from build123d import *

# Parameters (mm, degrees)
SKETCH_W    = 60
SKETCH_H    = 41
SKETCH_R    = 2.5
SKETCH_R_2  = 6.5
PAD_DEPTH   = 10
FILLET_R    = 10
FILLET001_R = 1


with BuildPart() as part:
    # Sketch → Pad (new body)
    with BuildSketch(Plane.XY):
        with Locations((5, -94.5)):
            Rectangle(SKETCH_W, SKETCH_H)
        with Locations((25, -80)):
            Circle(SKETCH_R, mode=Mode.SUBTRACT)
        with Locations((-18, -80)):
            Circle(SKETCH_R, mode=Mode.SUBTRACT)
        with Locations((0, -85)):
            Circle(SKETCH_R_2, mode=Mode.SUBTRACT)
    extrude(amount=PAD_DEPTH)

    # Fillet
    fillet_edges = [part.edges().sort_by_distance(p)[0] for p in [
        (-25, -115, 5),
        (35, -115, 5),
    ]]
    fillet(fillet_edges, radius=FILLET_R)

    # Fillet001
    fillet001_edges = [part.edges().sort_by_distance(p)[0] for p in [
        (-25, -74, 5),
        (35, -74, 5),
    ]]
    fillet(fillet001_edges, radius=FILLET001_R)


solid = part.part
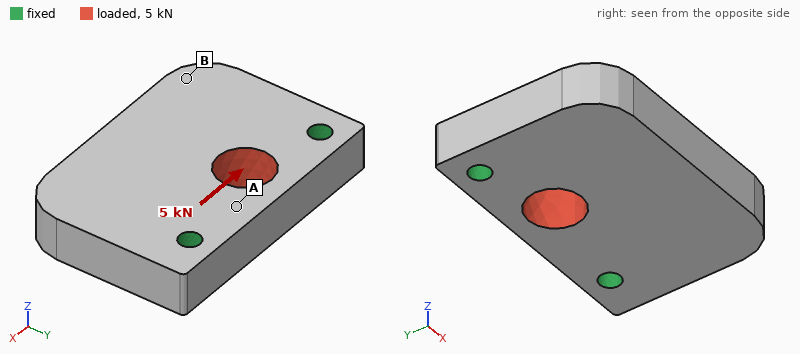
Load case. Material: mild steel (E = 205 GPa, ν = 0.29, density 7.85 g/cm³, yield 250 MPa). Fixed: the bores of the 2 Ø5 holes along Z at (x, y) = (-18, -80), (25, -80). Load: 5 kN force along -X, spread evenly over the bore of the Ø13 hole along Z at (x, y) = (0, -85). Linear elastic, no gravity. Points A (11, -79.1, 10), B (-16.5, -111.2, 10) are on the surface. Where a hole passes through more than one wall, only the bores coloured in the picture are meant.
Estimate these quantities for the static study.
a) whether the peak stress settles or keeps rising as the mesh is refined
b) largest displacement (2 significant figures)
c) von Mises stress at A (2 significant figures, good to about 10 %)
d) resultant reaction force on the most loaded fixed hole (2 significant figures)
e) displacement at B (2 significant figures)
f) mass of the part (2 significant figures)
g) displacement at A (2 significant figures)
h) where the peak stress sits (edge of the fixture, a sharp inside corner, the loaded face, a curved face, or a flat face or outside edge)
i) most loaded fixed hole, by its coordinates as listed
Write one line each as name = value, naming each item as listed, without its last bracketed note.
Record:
whether the peak stress settles or keeps rising as the mesh is refined = keeps rising
largest displacement = 2.1 µm
von Mises stress at A = 12 MPa
resultant reaction force on the most loaded fixed hole = 2.7 kN
displacement at B = 1.6 µm
mass of the part = 180 g
displacement at A = 0.88 µm
where the peak stress sits = edge of the fixture
most loaded fixed hole, by its coordinates as listed = (-18, -80)
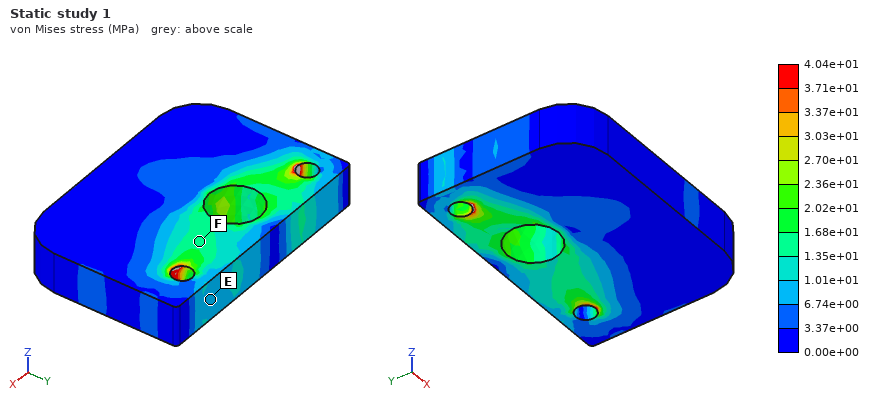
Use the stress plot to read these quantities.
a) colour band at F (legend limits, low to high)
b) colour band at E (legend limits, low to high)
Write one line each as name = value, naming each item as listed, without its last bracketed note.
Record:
colour band at F = 1.35e+01 to 1.68e+01 MPa
colour band at E = 6.74e+00 to 1.01e+01 MPa
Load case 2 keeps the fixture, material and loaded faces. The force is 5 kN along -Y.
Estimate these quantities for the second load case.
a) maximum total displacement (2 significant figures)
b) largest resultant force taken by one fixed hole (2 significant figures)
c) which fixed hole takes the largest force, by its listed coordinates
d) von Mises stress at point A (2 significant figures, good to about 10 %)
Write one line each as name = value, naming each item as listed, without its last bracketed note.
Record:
maximum total displacement = 4.4 µm
largest resultant force taken by one fixed hole = 3.0 kN
which fixed hole takes the largest force, by its listed coordinates = (-18, -80)
von Mises stress at point A = 11 MPa
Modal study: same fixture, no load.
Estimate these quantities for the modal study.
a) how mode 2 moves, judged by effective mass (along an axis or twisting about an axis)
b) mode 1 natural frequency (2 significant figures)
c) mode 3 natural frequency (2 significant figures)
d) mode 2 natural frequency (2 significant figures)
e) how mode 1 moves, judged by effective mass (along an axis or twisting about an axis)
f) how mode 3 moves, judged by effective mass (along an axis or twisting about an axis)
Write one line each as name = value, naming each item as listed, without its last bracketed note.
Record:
how mode 2 moves, judged by effective mass = twisting about Y
mode 1 natural frequency = 5300 Hz
mode 3 natural frequency = 16 kHz
mode 2 natural frequency = 10 kHz
how mode 1 moves, judged by effective mass = along Z
how mode 3 moves, judged by effective mass = along X
